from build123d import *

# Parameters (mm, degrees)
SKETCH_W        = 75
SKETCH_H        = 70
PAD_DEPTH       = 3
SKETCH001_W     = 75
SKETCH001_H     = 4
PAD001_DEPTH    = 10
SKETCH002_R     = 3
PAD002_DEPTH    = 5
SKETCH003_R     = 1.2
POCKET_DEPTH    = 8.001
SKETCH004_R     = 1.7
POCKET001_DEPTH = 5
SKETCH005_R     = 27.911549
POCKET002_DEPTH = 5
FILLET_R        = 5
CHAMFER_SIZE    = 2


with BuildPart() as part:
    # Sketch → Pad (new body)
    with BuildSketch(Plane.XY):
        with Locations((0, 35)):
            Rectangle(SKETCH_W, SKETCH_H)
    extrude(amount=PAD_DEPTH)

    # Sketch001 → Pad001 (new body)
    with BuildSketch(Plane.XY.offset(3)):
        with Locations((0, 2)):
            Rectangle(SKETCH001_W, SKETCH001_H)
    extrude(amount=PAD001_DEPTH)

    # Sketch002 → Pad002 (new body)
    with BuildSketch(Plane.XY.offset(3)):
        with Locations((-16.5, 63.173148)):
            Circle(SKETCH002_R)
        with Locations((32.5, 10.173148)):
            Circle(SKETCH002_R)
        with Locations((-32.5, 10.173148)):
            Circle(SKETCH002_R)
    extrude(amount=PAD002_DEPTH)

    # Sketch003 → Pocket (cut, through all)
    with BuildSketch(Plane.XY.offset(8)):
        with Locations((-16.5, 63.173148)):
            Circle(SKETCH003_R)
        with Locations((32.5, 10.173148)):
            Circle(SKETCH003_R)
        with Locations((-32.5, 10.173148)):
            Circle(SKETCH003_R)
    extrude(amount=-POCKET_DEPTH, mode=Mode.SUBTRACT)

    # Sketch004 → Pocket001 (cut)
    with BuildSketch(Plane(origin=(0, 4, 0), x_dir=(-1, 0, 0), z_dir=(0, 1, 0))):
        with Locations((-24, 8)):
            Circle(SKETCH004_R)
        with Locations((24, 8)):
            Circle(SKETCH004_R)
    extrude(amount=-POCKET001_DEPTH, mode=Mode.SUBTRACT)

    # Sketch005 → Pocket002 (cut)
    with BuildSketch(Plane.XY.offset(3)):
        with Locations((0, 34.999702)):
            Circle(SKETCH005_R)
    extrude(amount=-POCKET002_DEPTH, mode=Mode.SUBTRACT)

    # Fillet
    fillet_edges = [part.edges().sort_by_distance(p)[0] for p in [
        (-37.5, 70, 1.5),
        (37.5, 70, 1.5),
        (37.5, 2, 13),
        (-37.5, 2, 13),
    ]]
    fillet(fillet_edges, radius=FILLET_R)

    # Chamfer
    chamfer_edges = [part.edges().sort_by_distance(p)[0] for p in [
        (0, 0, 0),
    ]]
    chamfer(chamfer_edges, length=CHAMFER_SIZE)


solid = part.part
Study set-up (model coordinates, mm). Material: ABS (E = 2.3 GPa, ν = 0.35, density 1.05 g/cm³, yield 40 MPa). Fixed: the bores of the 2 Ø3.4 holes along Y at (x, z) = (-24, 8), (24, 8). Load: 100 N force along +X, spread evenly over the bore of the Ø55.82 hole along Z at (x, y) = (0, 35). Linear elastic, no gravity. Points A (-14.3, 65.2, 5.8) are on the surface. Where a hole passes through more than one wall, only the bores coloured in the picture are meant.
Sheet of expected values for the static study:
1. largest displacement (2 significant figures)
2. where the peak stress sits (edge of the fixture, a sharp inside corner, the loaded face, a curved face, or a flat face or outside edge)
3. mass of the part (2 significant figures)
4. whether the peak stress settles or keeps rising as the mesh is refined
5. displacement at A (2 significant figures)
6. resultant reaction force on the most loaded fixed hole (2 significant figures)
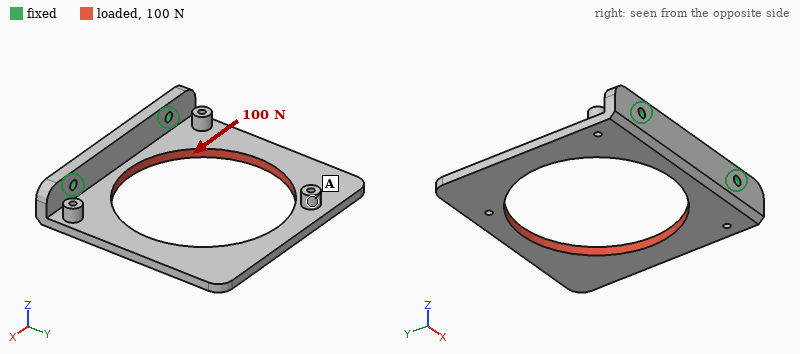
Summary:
0.74 mm
edge of the fixture
12 g
keeps rising
0.68 mm
76 N
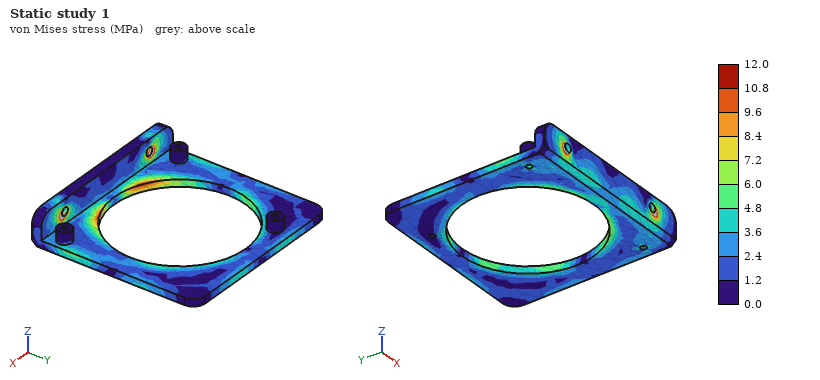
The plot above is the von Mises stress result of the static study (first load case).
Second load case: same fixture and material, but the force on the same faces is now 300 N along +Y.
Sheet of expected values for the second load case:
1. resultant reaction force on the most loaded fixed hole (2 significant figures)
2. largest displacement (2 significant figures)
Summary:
150 N
1.2 mm
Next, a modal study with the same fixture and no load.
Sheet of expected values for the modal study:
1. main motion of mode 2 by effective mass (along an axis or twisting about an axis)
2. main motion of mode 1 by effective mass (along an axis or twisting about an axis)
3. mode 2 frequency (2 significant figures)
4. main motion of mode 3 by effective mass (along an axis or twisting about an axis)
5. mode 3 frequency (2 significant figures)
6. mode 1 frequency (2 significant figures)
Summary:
twisting about Y
along Z
260 Hz
along X
700 Hz
120 Hz
